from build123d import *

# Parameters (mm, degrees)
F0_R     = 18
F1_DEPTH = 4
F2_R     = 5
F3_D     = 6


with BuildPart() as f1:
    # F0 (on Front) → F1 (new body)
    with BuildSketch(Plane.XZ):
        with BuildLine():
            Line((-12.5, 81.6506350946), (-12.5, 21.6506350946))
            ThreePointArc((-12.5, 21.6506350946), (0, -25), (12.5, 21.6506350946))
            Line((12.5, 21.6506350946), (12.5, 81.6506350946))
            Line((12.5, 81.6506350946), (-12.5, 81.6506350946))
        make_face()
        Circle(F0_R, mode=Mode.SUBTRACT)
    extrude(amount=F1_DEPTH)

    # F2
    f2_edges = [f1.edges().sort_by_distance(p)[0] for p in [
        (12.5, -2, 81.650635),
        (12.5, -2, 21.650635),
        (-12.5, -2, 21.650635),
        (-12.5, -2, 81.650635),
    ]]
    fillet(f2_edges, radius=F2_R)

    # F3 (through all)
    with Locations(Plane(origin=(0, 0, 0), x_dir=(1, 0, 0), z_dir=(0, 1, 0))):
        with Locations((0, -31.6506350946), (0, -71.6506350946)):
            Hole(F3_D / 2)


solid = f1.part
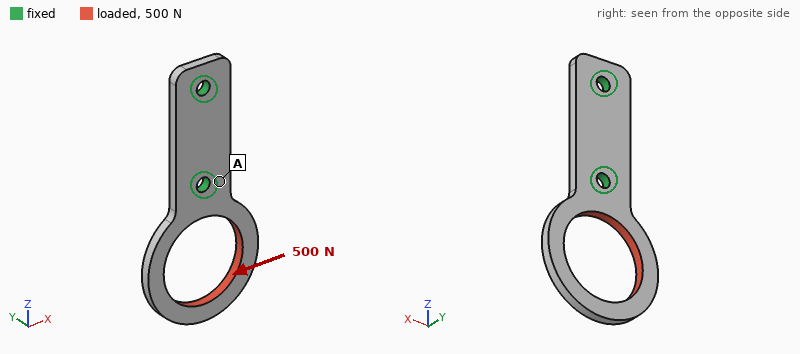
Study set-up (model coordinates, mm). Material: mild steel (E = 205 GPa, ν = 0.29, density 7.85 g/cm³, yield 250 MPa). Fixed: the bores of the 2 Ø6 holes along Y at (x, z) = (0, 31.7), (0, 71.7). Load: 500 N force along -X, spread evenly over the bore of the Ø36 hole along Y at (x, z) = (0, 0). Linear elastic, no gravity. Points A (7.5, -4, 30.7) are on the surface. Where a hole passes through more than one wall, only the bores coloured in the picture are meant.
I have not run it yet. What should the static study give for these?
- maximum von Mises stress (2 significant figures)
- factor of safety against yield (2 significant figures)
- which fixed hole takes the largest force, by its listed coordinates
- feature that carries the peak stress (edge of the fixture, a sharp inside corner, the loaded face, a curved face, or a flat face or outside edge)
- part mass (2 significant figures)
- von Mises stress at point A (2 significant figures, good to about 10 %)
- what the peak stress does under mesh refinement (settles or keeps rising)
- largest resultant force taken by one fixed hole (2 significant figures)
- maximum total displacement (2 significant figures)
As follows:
120 MPa
2.1
(0, 31.7)
a curved face
73 g
20 MPa
settles
750 N
75 µm
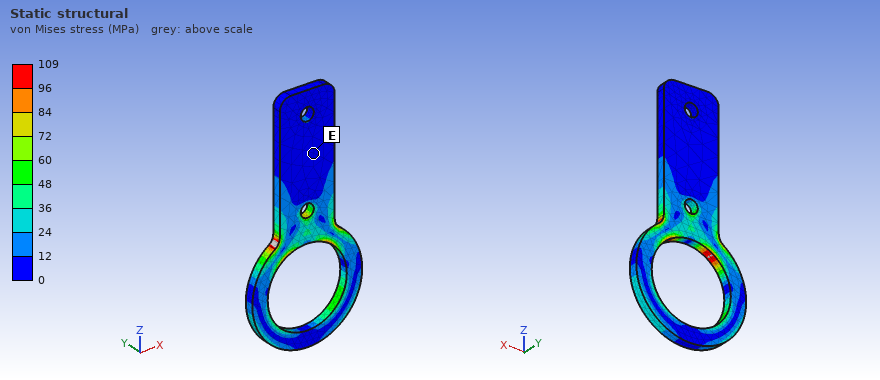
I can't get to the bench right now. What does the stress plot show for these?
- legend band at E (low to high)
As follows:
0 to 12 MPa
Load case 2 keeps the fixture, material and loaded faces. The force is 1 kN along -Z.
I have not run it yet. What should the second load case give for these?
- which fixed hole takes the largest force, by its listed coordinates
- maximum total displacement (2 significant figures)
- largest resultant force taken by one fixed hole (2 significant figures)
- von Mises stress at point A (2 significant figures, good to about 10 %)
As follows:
(0, 31.7)
18 µm
840 N
13 MPa
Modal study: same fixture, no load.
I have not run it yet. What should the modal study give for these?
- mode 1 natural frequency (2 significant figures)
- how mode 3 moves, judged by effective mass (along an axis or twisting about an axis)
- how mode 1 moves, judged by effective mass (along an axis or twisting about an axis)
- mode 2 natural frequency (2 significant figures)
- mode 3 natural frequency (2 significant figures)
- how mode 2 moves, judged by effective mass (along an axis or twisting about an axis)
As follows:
920 Hz
along X
along Y
2000 Hz
2600 Hz
twisting about Z
